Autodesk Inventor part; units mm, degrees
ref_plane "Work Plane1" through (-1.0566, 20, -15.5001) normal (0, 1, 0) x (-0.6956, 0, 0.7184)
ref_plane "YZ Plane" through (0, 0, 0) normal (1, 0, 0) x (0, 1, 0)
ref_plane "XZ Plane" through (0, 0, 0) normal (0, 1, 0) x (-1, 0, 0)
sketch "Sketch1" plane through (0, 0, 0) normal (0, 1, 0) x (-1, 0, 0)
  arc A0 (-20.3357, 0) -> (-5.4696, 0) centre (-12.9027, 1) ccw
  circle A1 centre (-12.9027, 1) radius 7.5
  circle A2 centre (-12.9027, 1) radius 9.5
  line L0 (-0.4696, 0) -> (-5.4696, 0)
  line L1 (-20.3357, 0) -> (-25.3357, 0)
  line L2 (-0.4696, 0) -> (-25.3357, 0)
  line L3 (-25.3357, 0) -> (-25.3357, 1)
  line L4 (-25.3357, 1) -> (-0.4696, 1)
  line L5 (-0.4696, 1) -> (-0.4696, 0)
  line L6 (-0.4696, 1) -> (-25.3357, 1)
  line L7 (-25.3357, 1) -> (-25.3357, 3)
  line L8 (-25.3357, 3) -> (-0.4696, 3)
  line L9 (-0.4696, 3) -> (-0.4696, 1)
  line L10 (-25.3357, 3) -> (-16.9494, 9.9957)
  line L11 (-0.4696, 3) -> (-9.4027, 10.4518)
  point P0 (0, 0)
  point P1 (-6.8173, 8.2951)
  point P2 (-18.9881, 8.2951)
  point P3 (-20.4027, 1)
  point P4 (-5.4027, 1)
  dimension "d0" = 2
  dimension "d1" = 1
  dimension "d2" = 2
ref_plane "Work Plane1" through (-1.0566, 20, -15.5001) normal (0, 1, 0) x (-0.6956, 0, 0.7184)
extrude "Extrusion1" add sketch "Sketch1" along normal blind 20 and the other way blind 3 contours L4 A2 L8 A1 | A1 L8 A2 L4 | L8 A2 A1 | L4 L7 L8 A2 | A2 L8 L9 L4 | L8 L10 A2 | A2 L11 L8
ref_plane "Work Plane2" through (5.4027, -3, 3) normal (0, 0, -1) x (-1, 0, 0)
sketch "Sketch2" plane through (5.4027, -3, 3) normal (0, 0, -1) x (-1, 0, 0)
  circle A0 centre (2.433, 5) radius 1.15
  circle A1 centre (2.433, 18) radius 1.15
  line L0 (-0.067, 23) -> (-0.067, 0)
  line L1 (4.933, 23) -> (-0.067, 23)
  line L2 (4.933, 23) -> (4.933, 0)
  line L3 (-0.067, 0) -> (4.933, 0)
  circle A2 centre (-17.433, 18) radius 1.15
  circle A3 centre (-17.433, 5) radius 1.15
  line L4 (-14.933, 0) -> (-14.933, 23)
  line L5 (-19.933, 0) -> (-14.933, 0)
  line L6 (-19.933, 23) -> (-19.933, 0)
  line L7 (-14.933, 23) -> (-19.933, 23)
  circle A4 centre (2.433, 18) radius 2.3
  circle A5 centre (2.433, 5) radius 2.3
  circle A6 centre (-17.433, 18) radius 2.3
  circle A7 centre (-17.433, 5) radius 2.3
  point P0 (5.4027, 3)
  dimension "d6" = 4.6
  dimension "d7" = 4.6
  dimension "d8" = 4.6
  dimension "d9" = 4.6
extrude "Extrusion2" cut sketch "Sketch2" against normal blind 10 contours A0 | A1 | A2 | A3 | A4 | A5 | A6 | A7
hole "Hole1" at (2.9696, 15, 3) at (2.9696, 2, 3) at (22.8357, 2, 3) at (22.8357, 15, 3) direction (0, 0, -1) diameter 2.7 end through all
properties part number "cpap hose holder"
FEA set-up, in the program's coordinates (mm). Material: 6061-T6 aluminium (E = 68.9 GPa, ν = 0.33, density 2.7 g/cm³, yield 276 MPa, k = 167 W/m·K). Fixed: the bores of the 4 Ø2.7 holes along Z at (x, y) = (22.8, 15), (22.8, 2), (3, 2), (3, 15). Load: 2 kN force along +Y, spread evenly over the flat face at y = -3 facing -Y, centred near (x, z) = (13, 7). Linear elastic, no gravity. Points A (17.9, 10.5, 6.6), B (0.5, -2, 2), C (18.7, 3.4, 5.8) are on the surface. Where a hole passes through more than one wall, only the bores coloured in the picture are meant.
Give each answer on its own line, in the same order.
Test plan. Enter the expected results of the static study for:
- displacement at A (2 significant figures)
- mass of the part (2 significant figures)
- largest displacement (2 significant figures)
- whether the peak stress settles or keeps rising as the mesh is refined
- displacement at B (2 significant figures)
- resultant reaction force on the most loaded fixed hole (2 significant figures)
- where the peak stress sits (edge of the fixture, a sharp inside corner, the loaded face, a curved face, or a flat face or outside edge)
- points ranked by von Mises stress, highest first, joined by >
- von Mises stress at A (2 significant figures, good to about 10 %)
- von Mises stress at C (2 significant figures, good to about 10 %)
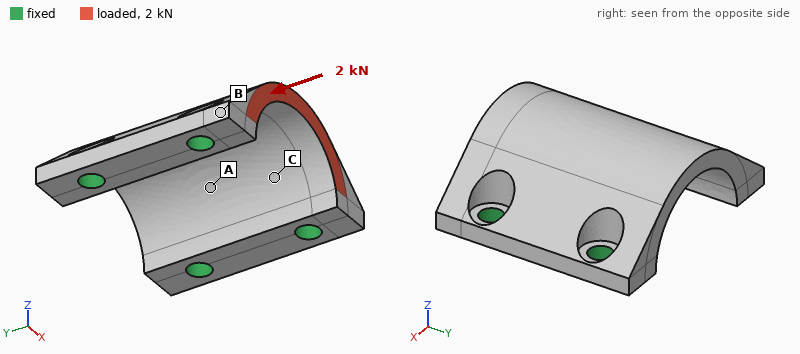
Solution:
7.7 µm
4.3 g
24 µm
keeps rising
6.0 µm
710 N
edge of the fixture
C > A > B
31 MPa
43 MPa
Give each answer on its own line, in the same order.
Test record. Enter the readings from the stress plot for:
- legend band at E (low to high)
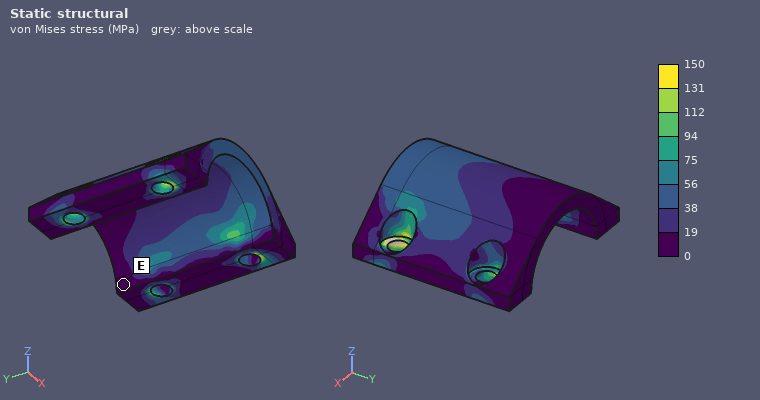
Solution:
0 to 19 MPa
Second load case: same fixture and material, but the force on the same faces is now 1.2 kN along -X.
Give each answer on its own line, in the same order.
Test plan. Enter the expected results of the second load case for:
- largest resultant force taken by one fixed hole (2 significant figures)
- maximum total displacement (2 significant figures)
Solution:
480 N
43 µm
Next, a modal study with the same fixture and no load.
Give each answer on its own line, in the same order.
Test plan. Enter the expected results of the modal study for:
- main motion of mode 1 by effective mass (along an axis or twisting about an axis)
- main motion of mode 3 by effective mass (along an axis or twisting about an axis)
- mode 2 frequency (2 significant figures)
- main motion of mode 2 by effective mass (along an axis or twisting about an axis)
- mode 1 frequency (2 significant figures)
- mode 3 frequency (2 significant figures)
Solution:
along X
twisting about Z
36 kHz
along Y
30 kHz
40 kHz
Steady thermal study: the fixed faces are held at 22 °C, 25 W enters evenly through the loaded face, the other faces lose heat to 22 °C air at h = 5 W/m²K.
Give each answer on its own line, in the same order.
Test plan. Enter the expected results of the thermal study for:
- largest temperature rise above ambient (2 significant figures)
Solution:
33 K
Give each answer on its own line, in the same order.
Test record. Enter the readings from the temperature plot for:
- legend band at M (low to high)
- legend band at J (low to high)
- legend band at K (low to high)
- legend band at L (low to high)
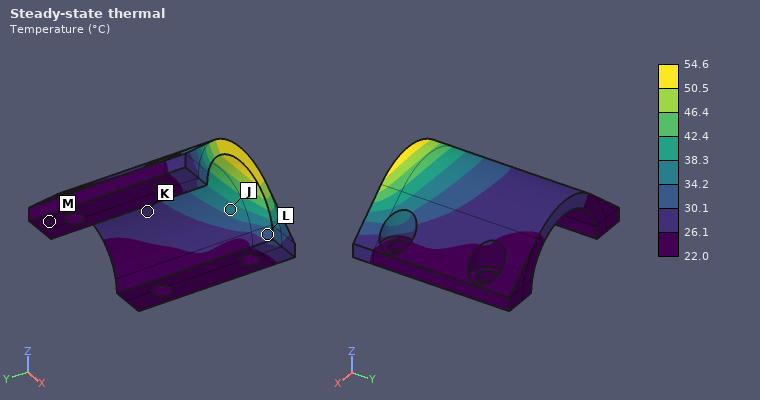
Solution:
22.0 to 26.1 °C
34.2 to 38.3 °C
26.1 to 30.1 °C
30.1 to 34.2 °C
